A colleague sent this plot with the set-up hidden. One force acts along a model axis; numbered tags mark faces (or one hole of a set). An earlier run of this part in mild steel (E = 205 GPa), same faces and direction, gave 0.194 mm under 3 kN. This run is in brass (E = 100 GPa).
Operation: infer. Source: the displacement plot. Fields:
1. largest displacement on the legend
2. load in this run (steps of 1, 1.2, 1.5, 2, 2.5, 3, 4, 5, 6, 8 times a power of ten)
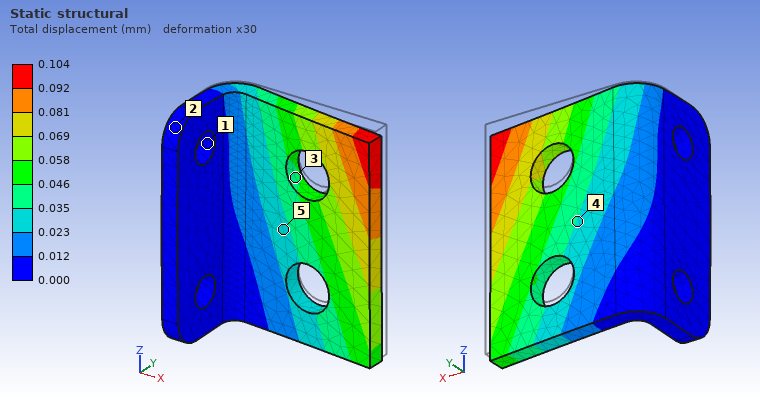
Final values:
0.104 mm
800 N
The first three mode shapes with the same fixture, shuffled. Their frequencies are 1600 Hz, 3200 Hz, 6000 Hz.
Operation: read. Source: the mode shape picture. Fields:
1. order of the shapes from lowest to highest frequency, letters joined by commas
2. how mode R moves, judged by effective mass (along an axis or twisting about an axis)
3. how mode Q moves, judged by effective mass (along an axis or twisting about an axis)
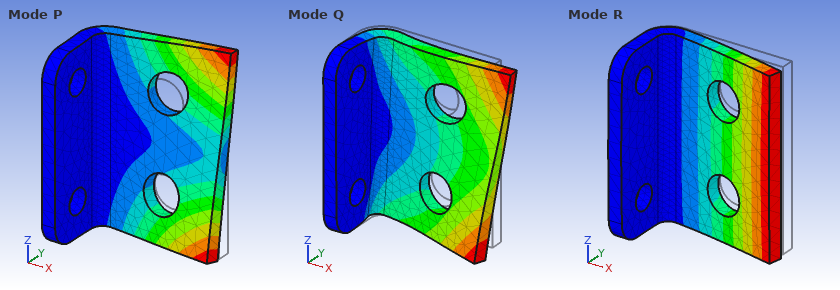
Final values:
R, P, Q
along Y
along Z
